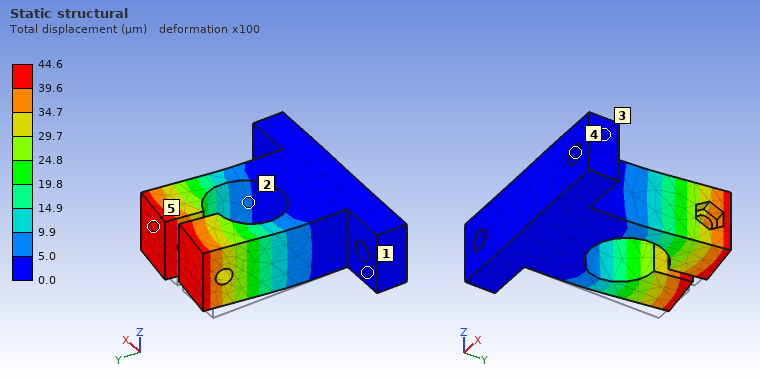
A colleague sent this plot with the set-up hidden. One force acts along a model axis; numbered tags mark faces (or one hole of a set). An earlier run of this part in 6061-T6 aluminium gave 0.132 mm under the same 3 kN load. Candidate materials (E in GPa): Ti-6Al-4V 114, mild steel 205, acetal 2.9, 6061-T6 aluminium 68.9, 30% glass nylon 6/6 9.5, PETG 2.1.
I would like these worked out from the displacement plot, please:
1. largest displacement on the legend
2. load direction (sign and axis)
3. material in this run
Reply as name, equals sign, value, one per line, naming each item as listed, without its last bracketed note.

largest displacement on the legend = 44.6 µm
load direction = +X
material in this run = mild steel
